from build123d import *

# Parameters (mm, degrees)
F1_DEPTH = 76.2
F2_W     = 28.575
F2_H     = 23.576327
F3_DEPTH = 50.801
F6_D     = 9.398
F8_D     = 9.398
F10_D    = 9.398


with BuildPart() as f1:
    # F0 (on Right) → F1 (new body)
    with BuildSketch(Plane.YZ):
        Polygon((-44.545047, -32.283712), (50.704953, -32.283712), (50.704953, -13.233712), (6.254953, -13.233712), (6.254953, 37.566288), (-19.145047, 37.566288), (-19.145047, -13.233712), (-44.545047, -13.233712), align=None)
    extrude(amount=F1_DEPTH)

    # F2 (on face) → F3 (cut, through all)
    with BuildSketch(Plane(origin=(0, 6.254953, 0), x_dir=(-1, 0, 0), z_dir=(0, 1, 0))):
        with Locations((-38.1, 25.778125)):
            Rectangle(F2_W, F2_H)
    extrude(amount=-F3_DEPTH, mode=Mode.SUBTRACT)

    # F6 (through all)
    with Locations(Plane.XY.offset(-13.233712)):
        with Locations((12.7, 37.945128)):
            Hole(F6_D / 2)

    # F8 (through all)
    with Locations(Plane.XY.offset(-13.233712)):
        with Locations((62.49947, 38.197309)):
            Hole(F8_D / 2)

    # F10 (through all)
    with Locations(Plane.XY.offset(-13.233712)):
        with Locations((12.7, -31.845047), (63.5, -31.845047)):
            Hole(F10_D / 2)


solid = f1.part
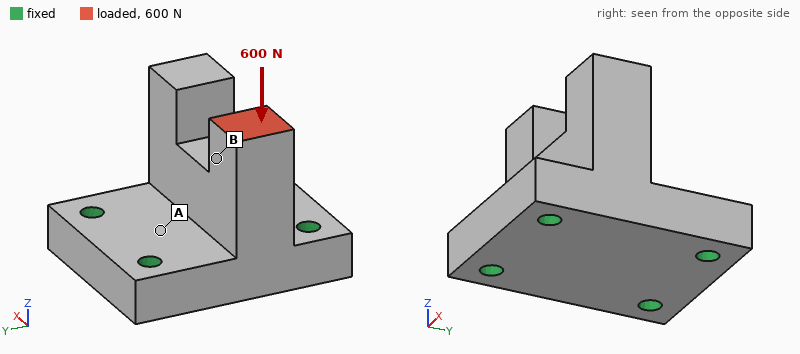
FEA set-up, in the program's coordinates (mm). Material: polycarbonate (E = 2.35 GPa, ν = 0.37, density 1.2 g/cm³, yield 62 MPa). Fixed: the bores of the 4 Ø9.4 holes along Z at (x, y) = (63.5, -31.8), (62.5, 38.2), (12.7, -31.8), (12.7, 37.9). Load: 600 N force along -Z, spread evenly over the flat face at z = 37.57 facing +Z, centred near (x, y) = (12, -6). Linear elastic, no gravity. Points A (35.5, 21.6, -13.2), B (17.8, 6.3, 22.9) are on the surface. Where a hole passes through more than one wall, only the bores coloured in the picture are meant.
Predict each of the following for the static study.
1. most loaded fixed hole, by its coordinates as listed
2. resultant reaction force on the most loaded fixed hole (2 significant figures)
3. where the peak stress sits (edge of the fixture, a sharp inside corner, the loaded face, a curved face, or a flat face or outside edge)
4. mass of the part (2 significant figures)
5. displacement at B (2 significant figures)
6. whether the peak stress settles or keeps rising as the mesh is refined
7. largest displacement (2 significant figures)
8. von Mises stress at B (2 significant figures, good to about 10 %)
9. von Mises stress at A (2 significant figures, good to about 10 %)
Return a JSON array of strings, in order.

["(12.7, -31.8)", "390 N", "edge of the fixture", "260 g", "47 µm", "keeps rising", "72 µm", "0.95 MPa", "0.32 MPa"]
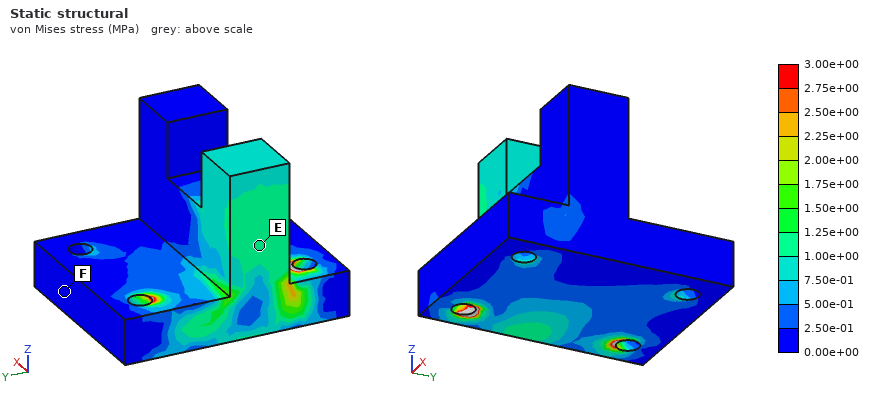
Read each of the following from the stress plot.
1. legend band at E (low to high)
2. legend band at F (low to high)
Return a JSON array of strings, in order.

["1.00e+00 to 1.25e+00 MPa", "0.00e+00 to 2.50e-01 MPa"]
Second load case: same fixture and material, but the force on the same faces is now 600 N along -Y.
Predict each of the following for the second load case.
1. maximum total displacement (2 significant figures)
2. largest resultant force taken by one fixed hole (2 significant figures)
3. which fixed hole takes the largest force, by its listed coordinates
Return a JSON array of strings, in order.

["0.46 mm", "510 N", "(12.7, -31.8)"]
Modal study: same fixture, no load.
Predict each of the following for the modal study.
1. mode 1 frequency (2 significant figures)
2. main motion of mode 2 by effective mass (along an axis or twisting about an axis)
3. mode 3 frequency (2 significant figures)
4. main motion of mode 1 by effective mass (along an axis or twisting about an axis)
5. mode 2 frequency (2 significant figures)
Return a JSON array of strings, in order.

["1500 Hz", "along X", "2000 Hz", "along Y", "1700 Hz"]
